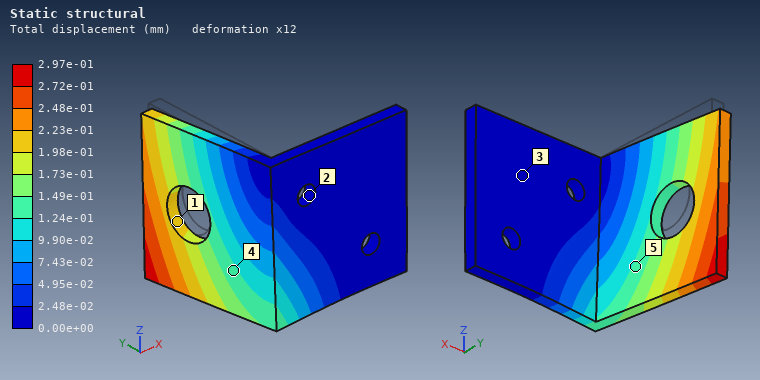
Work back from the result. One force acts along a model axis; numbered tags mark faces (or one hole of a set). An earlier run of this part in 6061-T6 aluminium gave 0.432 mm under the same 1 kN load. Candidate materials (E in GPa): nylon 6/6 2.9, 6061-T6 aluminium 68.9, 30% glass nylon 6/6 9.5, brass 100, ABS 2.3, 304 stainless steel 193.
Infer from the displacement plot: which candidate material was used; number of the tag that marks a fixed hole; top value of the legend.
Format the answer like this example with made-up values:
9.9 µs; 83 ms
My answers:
brass; 2; 2.97e-01 mm
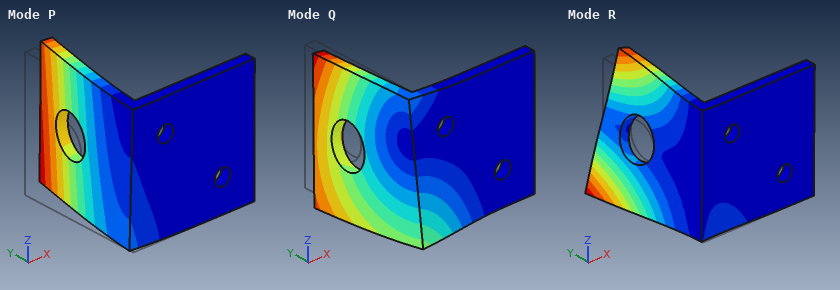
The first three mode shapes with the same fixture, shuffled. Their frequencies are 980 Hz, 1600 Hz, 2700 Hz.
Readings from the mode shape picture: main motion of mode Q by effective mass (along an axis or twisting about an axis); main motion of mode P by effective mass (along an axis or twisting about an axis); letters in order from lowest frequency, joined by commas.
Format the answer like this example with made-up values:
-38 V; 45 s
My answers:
along Z; along X; P, Q, R
